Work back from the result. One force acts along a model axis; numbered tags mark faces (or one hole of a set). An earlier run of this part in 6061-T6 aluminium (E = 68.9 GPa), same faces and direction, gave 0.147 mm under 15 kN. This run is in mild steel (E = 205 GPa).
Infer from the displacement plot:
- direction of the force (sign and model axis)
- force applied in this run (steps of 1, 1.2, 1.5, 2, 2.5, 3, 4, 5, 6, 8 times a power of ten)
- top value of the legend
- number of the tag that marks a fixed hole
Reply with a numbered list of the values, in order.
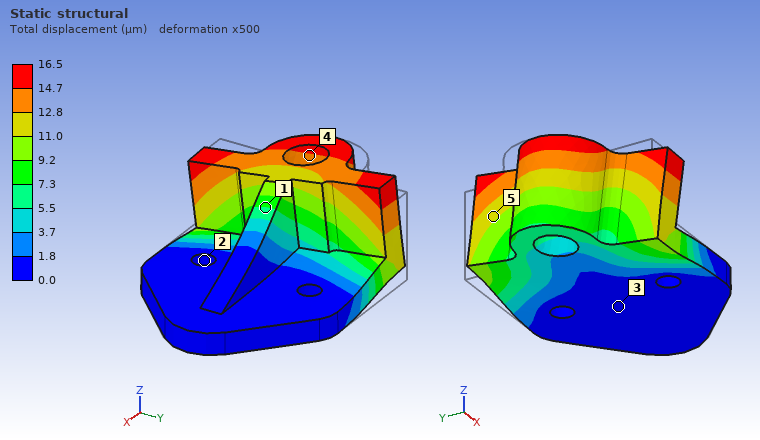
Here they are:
1. -Y
2. 5 kN
3. 16.5 µm
4. 2
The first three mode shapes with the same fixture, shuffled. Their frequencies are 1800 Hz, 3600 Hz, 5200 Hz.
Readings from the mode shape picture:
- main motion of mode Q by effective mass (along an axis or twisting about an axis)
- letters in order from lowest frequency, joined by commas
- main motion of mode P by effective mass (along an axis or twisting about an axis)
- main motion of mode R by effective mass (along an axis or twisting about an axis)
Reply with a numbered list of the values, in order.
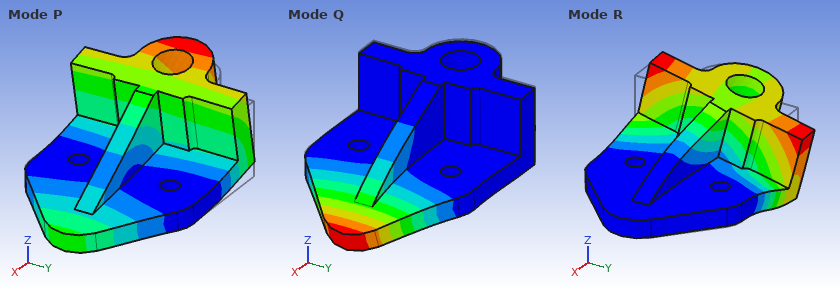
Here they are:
1. along Z
2. P, R, Q
3. along Z
4. along Y
